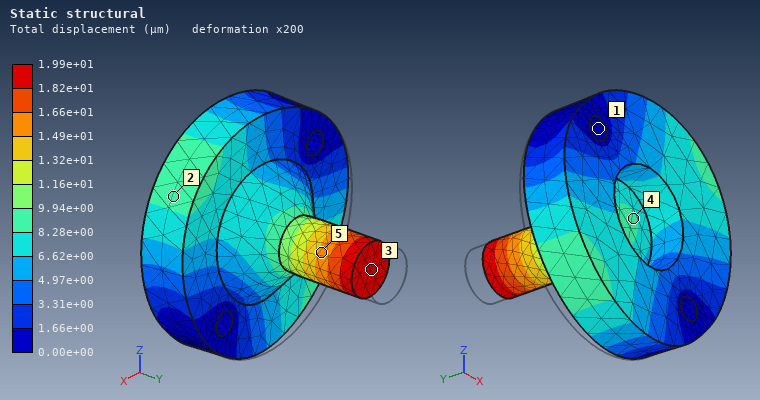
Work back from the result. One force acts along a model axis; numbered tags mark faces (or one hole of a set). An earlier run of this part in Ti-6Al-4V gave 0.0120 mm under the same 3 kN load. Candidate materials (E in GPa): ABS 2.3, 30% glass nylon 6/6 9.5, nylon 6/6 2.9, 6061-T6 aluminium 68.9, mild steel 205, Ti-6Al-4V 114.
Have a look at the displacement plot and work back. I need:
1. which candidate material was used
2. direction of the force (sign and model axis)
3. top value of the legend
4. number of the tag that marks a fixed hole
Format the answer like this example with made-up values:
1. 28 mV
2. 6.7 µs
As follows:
1. 6061-T6 aluminium
2. -Y
3. 1.99e+01 µm
4. 1
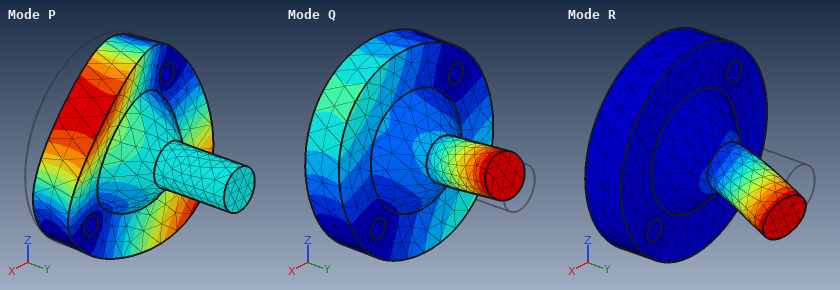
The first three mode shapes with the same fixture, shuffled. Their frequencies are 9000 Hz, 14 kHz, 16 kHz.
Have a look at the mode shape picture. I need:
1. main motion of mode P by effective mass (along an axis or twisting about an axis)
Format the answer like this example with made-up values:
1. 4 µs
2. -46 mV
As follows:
1. along Y
